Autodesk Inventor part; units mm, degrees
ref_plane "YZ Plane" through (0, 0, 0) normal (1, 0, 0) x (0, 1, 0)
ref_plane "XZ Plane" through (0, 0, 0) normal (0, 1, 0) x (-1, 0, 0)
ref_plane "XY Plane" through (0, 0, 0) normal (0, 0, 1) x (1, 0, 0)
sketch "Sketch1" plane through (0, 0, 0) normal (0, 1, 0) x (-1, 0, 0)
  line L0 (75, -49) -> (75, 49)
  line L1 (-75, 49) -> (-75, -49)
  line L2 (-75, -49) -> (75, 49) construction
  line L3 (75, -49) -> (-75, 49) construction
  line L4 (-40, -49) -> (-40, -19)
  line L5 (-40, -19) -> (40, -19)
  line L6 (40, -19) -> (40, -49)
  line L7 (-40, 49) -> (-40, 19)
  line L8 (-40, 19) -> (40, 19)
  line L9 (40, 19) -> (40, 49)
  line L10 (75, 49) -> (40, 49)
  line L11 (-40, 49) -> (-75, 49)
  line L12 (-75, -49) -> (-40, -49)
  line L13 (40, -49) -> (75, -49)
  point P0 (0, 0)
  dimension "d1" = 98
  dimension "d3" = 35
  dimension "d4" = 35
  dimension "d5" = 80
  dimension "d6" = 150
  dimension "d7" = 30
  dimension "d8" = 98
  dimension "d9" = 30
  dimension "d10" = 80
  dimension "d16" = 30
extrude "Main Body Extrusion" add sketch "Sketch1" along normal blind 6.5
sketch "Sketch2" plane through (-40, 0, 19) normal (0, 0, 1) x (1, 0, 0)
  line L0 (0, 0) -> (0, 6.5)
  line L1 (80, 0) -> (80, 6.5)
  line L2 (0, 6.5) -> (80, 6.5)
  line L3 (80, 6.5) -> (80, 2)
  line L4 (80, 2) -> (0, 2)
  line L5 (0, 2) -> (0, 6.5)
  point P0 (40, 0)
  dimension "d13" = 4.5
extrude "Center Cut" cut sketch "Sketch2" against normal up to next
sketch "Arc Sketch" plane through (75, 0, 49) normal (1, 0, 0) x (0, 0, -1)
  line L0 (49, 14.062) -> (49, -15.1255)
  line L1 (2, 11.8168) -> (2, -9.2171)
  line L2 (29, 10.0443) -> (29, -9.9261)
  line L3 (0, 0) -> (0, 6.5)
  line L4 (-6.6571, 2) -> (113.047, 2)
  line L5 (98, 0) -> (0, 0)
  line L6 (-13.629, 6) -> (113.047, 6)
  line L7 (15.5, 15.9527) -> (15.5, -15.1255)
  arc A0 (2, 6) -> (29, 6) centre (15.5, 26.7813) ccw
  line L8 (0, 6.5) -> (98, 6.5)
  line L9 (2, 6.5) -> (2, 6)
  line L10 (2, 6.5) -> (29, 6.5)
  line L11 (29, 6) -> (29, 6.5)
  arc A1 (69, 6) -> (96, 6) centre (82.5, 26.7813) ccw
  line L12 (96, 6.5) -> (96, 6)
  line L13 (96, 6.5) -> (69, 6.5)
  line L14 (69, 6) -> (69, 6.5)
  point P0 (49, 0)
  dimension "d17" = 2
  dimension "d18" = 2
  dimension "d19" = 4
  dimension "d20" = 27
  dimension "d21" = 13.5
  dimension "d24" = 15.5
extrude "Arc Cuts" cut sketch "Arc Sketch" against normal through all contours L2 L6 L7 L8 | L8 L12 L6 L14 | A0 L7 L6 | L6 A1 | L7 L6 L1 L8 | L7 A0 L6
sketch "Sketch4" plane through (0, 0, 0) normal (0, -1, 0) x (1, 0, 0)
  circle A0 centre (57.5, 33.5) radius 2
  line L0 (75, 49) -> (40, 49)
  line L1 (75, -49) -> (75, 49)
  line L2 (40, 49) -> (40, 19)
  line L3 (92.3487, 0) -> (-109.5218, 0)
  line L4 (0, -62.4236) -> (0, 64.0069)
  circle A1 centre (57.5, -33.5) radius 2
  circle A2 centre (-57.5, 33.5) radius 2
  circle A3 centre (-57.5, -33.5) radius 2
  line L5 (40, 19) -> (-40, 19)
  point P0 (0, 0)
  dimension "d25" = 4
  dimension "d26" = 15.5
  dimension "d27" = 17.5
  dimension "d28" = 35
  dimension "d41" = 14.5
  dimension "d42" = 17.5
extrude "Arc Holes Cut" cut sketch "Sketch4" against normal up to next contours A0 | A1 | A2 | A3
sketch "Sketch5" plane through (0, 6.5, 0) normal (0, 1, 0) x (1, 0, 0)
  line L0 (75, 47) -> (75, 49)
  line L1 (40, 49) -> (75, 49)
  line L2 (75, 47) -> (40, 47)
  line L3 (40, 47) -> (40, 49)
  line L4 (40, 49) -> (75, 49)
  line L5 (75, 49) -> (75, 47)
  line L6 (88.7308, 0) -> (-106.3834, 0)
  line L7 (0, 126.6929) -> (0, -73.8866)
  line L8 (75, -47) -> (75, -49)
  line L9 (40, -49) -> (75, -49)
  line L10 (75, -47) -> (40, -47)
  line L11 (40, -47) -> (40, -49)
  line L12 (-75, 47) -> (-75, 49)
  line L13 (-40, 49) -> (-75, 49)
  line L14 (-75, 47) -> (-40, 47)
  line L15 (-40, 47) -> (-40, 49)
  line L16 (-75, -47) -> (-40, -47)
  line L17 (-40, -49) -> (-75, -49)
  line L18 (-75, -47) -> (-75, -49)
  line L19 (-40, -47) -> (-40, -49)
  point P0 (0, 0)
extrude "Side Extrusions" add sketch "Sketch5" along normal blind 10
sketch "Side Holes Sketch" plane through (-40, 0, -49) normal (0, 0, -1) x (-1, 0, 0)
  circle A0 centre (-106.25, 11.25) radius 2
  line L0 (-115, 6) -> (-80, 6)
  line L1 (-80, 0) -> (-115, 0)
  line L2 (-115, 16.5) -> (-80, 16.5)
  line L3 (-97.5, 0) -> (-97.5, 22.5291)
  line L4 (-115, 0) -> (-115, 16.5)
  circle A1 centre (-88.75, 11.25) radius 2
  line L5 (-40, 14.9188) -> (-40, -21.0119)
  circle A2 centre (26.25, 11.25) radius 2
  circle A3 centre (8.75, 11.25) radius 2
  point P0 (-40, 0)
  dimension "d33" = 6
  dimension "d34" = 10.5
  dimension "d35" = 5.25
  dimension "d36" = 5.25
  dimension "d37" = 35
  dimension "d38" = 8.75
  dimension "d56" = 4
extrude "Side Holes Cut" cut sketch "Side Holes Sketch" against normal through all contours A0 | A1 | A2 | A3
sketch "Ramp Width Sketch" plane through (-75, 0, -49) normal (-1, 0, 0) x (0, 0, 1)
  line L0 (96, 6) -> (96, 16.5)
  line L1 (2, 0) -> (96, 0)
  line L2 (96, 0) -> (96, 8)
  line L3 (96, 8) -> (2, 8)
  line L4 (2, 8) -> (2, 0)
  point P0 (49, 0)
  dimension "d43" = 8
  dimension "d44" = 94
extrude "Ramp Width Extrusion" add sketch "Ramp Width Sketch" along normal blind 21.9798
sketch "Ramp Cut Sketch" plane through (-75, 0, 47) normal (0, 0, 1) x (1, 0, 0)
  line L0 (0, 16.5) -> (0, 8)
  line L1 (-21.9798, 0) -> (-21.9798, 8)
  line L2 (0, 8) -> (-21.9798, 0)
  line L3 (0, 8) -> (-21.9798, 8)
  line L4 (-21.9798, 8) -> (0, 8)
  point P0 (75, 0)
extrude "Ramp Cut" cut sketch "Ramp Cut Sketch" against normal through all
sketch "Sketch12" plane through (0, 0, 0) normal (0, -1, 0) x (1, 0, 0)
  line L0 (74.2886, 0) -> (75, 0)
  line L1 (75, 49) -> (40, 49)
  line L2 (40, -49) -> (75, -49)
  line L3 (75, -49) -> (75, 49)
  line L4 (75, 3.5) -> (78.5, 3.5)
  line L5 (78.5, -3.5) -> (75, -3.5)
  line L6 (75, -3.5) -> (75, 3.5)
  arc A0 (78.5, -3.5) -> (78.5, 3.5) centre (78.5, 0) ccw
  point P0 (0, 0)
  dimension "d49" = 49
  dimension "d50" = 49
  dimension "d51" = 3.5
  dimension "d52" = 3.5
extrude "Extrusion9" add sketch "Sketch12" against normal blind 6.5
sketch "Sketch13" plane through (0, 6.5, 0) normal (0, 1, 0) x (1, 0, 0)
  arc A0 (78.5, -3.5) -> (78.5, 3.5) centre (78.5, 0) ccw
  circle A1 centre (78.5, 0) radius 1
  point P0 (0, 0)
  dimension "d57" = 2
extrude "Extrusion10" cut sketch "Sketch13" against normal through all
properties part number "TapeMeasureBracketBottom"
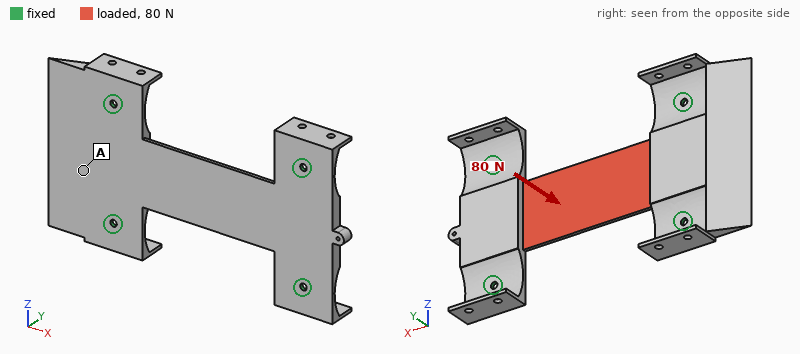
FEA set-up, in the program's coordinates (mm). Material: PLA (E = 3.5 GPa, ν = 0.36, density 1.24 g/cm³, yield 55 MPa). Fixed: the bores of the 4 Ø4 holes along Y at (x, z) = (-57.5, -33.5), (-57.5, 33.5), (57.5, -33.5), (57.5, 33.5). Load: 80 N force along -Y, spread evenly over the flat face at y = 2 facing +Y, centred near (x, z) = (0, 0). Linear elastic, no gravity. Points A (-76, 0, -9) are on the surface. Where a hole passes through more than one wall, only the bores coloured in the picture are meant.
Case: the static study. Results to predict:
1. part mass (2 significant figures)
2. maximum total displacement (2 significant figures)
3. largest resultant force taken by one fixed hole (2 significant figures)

61 g
2.3 mm
73 N
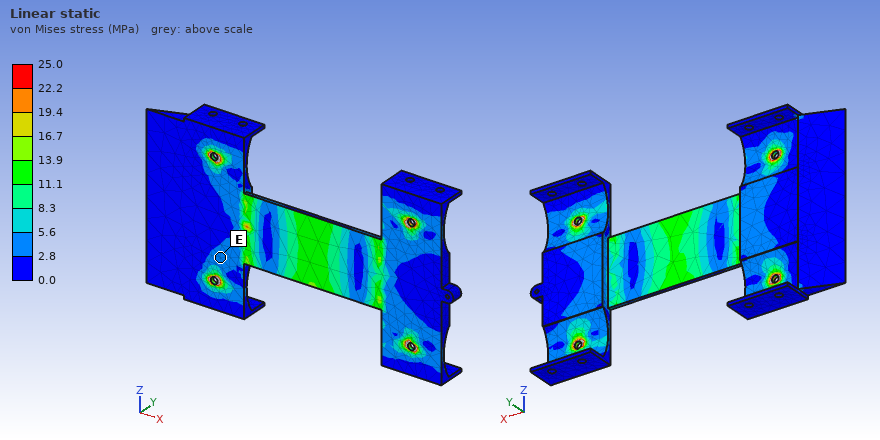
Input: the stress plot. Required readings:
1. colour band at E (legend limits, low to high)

2.8 to 5.6 MPa
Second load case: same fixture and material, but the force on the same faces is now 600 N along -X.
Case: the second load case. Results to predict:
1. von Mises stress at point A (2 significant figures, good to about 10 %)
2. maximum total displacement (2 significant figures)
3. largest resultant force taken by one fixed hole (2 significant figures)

0.85 MPa
0.12 mm
160 N
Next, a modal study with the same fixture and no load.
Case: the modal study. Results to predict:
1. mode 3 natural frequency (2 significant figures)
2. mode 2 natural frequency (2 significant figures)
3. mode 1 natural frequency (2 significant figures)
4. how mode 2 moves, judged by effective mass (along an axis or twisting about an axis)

810 Hz
490 Hz
340 Hz
along Y
